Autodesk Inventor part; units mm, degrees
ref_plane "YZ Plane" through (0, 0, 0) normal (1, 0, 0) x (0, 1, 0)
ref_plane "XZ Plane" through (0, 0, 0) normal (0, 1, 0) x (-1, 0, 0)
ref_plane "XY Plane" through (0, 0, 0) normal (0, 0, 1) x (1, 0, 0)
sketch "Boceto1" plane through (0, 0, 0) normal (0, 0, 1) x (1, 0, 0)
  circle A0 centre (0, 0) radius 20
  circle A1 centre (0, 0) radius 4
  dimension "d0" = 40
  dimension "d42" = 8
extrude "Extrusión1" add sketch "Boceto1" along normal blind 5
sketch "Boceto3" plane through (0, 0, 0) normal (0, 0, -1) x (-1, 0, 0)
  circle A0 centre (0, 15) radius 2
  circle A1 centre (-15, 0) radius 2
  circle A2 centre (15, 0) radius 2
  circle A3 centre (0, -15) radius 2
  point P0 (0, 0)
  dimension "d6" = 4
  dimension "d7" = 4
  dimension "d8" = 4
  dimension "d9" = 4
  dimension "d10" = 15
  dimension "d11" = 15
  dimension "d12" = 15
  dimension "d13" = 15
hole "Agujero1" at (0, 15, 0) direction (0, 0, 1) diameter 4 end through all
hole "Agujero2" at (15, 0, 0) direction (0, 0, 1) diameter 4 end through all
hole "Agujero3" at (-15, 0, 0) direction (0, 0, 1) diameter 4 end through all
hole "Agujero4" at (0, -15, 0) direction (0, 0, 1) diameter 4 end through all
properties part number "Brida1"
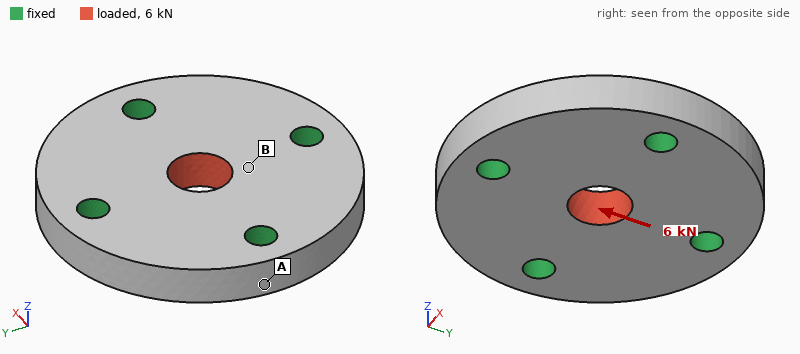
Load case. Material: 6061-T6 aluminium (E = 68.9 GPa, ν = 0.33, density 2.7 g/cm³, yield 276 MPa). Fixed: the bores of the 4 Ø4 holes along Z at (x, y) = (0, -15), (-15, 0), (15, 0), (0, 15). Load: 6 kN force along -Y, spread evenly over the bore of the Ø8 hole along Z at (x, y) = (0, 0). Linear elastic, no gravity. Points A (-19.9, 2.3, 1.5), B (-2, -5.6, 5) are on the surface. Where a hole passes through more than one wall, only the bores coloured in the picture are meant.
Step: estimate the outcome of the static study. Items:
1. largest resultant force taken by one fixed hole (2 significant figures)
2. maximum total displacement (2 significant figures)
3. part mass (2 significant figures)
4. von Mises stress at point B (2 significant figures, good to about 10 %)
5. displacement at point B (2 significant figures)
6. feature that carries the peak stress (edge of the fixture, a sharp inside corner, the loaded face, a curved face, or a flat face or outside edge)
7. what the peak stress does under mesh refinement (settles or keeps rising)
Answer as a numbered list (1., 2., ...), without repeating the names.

1. 2.0 kN
2. 7.9 µm
3. 16 g
4. 51 MPa
5. 5.7 µm
6. edge of the fixture
7. keeps rising
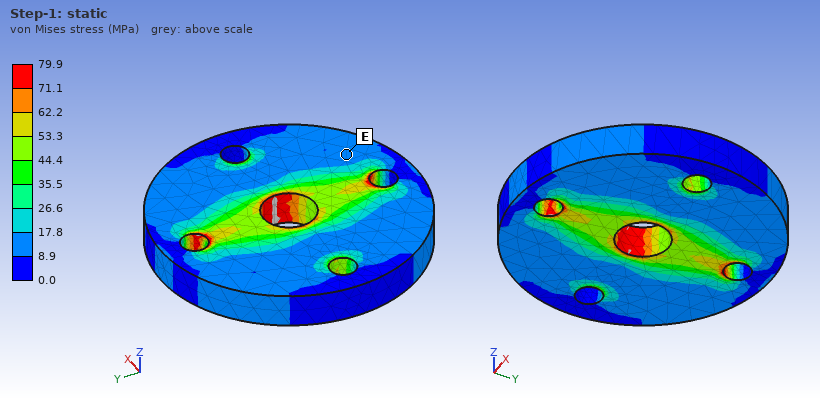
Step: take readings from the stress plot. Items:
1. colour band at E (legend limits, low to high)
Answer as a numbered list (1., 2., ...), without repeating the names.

1. 8.9 to 17.8 MPa
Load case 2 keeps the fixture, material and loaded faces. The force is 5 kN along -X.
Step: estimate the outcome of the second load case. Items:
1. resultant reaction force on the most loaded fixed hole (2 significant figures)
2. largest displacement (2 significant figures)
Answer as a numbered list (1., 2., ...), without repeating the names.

1. 1.7 kN
2. 6.6 µm
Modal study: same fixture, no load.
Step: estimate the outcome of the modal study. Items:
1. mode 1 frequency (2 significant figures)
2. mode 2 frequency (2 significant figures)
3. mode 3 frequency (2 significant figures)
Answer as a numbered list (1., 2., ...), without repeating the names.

1. 35 kHz
2. 37 kHz
3. 37 kHz
